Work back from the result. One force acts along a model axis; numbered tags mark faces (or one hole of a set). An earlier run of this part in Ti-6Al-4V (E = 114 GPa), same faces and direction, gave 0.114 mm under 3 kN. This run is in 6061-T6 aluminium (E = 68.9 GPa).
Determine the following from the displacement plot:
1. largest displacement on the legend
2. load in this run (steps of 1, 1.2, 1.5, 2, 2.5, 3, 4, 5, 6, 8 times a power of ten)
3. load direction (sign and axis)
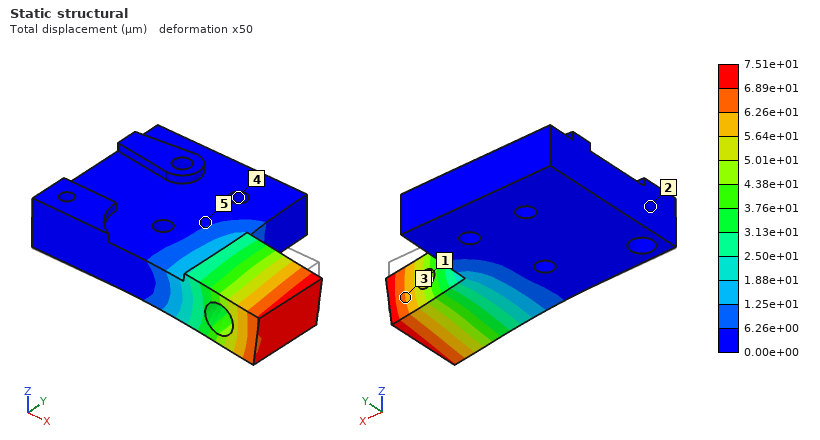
7.51e+01 µm
1.2 kN
-Z
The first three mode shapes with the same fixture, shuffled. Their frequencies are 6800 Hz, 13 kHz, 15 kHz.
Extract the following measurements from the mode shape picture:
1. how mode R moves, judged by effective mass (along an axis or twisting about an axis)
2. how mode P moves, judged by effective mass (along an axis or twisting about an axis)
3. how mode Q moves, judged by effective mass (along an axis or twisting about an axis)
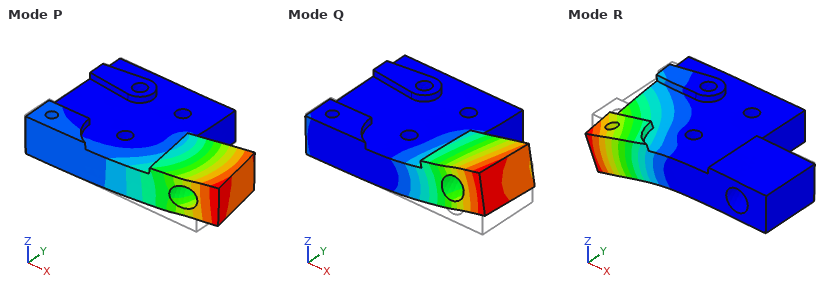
along Z
along Y
along Z
